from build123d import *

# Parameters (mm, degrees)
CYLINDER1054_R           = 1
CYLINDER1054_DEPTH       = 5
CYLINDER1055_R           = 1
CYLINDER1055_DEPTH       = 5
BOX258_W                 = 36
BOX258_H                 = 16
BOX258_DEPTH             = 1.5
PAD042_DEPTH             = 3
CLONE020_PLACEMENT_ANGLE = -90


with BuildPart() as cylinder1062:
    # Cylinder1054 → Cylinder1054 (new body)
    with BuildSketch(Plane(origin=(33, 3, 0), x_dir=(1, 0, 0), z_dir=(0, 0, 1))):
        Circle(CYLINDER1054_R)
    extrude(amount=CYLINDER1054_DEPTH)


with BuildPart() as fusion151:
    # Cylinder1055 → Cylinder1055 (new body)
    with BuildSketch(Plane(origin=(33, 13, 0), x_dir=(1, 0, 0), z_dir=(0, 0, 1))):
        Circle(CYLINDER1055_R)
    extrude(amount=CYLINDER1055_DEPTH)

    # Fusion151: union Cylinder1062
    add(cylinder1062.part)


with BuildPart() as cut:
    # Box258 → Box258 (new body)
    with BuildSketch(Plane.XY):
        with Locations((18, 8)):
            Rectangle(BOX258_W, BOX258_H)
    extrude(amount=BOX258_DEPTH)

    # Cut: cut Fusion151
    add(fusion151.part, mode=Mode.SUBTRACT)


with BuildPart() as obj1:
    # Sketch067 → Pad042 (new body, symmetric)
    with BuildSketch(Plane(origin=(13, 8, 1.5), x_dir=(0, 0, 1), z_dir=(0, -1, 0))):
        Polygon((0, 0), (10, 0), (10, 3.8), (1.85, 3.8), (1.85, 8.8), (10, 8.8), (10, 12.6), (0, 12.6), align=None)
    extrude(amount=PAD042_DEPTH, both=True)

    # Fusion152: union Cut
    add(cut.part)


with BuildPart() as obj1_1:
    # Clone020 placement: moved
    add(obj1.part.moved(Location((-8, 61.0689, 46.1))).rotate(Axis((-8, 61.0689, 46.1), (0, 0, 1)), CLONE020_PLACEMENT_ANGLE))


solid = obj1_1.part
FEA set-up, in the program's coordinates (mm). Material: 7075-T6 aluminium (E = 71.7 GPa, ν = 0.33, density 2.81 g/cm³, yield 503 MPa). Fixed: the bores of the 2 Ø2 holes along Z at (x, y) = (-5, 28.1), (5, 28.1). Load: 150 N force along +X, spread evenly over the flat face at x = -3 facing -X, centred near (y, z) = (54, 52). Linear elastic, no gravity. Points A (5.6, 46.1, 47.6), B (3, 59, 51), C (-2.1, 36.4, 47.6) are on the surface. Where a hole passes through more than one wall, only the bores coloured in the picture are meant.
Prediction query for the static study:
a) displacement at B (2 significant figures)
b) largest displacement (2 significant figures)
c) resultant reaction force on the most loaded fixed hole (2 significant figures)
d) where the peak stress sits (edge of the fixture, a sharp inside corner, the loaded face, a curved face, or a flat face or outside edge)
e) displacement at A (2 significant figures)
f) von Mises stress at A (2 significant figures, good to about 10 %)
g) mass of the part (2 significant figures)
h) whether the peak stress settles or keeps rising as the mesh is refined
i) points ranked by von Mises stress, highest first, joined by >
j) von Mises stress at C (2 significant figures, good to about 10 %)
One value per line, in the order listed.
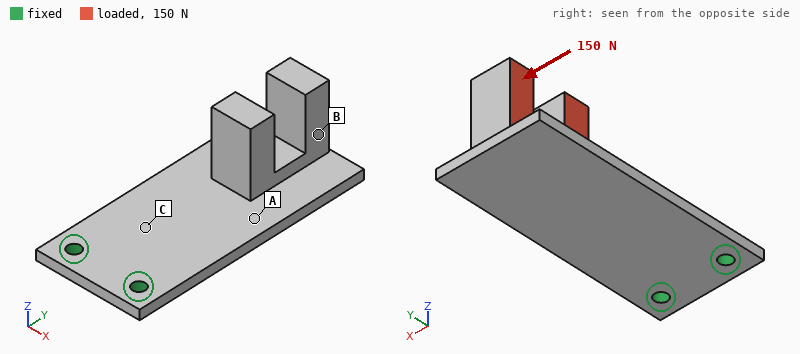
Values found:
0.18 mm
0.36 mm
370 N
edge of the fixture
0.13 mm
96 MPa
3.8 g
keeps rising
C > A > B
120 MPa
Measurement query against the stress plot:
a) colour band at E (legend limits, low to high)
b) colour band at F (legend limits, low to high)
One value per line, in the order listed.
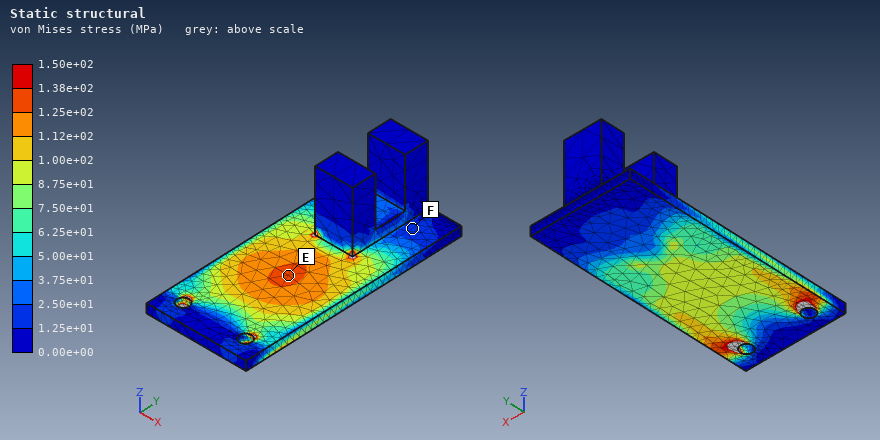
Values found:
1.25e+02 to 1.38e+02 MPa
1.25e+01 to 2.50e+01 MPa
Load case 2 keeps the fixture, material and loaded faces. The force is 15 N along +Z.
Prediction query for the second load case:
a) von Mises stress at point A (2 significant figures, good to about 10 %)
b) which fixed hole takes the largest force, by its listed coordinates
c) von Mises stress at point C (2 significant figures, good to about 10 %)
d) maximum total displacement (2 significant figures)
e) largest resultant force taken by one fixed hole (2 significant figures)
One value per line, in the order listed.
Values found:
21 MPa
(-5, 28.1)
43 MPa
0.40 mm
11 N
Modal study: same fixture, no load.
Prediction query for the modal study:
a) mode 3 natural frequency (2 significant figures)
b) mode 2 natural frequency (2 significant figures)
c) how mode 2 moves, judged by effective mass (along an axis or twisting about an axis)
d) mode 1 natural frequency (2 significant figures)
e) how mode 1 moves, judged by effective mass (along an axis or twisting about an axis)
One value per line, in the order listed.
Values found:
4800 Hz
2900 Hz
along X
720 Hz
along Z
